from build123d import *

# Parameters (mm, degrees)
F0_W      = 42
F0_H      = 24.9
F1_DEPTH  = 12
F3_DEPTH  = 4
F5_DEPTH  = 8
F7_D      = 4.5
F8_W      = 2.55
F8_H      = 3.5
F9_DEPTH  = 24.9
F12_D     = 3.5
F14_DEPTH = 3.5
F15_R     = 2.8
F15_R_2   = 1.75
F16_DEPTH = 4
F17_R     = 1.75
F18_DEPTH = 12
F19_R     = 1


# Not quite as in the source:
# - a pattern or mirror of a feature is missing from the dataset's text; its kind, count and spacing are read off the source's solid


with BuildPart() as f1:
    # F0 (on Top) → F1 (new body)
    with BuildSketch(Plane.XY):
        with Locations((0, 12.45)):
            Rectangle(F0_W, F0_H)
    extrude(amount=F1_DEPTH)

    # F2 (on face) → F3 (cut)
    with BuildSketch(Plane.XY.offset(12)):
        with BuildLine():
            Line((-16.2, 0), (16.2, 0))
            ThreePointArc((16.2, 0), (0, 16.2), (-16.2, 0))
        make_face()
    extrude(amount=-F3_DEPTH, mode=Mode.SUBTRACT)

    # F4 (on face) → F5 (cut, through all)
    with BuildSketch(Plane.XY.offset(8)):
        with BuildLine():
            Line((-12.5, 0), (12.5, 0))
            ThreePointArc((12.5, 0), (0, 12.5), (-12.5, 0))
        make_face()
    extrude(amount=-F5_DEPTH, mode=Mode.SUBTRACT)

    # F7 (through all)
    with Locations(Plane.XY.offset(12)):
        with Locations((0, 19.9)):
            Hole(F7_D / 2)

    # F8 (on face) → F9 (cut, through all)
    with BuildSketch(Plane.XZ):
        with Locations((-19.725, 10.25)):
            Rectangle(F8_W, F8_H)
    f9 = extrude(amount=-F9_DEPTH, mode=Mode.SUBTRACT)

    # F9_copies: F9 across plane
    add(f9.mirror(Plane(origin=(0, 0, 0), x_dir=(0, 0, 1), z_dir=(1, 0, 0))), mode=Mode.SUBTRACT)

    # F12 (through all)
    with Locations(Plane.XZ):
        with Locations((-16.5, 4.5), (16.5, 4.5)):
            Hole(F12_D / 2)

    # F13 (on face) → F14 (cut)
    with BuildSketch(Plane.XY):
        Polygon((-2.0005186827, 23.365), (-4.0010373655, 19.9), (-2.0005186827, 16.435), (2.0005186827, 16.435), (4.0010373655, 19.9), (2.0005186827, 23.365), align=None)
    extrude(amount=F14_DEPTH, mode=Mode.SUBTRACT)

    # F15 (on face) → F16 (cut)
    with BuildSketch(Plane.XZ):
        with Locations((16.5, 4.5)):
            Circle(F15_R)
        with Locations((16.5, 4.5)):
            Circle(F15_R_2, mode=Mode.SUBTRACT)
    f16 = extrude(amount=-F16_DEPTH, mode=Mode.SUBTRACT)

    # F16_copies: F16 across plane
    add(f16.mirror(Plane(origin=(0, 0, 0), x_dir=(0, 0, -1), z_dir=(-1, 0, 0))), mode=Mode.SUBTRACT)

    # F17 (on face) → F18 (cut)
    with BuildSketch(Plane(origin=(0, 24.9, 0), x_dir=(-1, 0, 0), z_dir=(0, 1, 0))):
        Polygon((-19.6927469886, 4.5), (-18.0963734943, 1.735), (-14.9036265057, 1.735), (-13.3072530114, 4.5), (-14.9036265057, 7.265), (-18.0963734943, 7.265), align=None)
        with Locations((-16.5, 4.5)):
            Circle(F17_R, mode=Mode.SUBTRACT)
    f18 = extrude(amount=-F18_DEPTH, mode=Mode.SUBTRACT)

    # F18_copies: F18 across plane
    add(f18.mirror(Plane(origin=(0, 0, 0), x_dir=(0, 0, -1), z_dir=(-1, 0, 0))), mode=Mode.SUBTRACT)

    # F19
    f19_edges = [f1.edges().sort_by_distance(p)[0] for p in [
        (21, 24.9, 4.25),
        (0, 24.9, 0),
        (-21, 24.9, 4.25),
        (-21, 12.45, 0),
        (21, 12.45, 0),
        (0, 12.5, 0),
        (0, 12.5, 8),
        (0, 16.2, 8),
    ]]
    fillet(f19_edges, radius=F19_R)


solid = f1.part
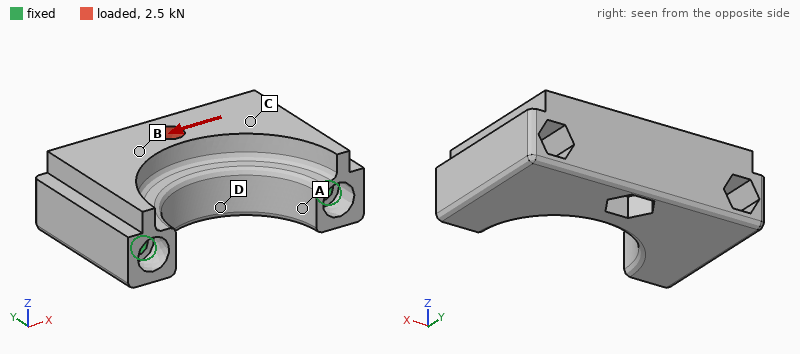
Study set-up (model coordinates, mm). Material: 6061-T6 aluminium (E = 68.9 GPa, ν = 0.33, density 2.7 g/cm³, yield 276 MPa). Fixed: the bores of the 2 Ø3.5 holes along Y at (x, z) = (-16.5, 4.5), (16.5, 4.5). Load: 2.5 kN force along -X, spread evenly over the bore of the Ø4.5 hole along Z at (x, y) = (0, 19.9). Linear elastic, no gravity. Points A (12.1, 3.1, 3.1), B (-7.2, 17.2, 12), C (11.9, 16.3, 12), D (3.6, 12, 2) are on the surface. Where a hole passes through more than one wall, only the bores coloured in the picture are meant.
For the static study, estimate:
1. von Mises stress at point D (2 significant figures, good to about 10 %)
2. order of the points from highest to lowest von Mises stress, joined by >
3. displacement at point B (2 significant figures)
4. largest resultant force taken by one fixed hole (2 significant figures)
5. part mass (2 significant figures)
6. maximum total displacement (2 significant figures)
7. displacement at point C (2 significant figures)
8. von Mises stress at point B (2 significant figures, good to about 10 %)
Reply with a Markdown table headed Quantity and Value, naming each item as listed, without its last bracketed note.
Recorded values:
| Quantity | Value |
|---|---|
| von Mises stress at point D | 25 MPa |
| order of the points from highest to lowest von Mises stress, joined by > | D > B > C > A |
| displacement at point B | 5.8 µm |
| largest resultant force taken by one fixed hole | 1.4 kN |
| part mass | 19 g |
| maximum total displacement | 8.6 µm |
| displacement at point C | 4.7 µm |
| von Mises stress at point B | 17 MPa |
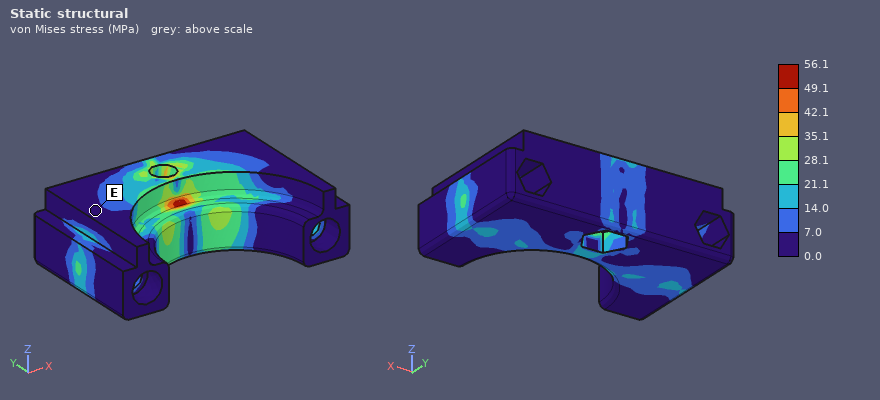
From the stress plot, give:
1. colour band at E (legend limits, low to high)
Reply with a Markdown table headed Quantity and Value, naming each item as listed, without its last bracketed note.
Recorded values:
| Quantity | Value |
|---|---|
| colour band at E | 0.0 to 7.0 MPa |
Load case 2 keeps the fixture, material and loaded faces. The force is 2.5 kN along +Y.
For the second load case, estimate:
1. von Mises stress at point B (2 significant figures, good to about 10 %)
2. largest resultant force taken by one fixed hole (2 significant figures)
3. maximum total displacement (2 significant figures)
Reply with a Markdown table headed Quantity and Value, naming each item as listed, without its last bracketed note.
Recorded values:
| Quantity | Value |
|---|---|
| von Mises stress at point B | 25 MPa |
| largest resultant force taken by one fixed hole | 1.6 kN |
| maximum total displacement | 21 µm |
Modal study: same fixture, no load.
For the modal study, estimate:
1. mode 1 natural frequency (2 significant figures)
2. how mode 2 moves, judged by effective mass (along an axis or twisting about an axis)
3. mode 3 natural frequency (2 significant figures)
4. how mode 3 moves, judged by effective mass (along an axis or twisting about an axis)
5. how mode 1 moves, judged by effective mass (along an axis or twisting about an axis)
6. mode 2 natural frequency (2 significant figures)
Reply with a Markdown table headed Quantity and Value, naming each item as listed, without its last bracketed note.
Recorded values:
| Quantity | Value |
|---|---|
| mode 1 natural frequency | 14 kHz |
| how mode 2 moves, judged by effective mass | twisting about Y |
| mode 3 natural frequency | 31 kHz |
| how mode 3 moves, judged by effective mass | along X |
| how mode 1 moves, judged by effective mass | along Z |
| mode 2 natural frequency | 26 kHz |
